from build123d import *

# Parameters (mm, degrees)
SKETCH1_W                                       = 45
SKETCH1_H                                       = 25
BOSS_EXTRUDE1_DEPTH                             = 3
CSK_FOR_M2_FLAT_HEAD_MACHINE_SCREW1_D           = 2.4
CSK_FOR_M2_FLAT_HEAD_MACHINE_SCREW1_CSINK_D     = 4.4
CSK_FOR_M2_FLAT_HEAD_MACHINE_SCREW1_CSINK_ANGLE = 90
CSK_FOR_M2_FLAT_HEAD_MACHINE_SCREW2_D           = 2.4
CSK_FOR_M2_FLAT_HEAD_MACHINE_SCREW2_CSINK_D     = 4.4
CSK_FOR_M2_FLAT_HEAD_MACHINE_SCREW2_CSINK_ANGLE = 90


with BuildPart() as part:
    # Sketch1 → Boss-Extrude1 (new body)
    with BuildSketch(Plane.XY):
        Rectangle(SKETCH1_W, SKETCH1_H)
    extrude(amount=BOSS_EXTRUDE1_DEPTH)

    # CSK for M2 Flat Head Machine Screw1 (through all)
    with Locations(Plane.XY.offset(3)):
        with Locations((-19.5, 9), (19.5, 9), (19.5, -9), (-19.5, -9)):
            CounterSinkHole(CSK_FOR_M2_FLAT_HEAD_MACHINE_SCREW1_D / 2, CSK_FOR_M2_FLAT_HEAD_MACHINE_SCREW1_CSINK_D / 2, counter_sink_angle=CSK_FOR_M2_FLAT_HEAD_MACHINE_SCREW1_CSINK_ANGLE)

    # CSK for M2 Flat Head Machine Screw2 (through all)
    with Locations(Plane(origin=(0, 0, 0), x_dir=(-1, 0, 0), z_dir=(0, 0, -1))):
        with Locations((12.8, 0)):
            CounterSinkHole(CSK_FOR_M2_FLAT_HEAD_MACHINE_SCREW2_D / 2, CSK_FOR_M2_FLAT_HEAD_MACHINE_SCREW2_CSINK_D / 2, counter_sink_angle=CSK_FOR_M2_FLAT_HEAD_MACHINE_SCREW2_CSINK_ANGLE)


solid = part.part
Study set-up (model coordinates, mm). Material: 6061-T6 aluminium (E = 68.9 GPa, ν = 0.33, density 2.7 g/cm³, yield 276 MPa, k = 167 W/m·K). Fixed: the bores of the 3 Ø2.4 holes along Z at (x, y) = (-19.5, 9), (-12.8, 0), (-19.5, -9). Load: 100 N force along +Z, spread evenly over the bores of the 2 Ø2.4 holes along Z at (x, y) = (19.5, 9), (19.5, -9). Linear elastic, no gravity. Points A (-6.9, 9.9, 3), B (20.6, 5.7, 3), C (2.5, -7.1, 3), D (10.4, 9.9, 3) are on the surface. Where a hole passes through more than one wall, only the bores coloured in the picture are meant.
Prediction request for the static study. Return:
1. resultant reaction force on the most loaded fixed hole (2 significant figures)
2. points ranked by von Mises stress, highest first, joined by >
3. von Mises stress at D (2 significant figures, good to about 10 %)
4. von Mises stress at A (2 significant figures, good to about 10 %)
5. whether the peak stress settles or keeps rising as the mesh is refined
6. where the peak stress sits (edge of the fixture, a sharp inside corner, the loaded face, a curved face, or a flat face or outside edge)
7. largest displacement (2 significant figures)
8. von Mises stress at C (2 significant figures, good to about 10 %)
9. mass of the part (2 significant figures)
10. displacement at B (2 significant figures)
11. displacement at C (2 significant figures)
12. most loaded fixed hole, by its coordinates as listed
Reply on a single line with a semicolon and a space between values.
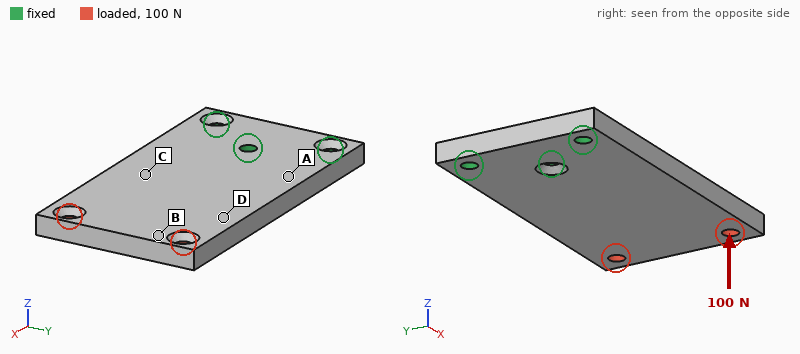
360 N; A > C > D > B; 25 MPa; 64 MPa; keeps rising; edge of the fixture; 0.38 mm; 43 MPa; 8.9 g; 0.35 mm; 0.11 mm; (-12.8, 0)
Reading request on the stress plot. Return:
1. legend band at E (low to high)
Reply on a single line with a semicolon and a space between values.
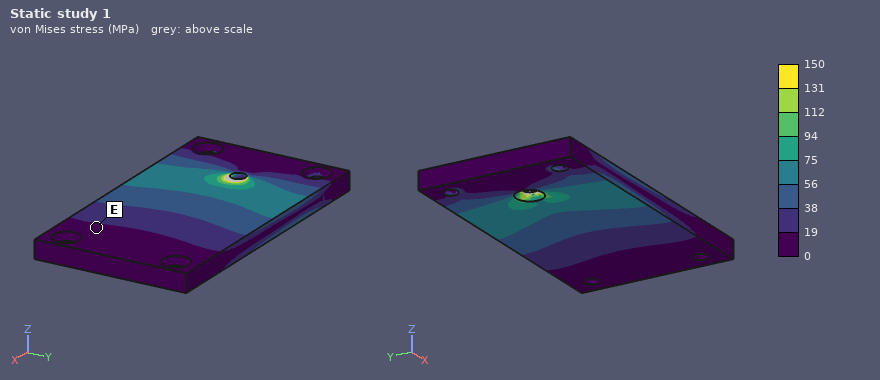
0 to 19 MPa
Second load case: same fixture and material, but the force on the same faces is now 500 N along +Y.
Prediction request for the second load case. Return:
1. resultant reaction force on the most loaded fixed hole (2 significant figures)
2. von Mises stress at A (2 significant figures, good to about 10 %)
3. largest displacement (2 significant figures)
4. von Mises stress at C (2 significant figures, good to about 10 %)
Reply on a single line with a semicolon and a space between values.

790 N; 33 MPa; 64 µm; 16 MPa
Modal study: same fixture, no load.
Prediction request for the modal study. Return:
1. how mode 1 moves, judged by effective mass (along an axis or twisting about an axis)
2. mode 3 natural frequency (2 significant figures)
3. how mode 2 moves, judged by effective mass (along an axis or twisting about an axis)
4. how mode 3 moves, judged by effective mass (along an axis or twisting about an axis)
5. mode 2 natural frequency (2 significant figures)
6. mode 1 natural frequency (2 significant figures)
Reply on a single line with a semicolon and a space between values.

along Z; 9800 Hz; twisting about X; along Y; 5100 Hz; 1800 Hz
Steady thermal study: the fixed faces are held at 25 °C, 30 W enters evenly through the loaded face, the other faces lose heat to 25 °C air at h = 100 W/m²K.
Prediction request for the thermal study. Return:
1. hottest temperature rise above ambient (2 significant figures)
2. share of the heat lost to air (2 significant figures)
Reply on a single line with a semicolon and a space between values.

80 K; 27 %
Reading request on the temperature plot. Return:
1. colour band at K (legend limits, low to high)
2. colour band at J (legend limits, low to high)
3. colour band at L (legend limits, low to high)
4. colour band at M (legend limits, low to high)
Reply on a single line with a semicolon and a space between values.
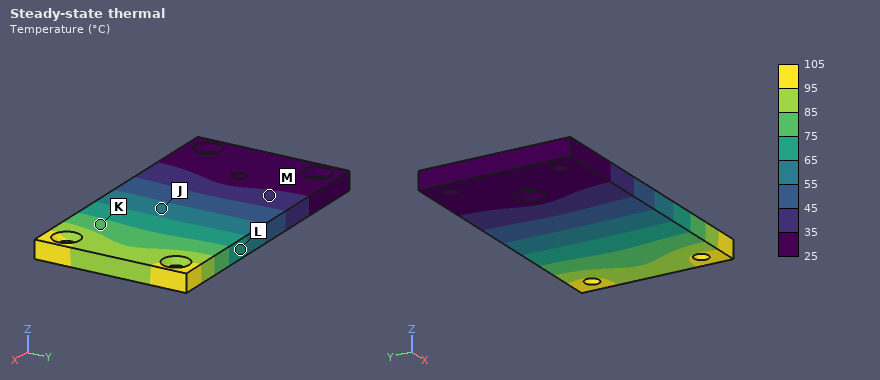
75 to 85 °C; 55 to 65 °C; 65 to 75 °C; 35 to 45 °C
